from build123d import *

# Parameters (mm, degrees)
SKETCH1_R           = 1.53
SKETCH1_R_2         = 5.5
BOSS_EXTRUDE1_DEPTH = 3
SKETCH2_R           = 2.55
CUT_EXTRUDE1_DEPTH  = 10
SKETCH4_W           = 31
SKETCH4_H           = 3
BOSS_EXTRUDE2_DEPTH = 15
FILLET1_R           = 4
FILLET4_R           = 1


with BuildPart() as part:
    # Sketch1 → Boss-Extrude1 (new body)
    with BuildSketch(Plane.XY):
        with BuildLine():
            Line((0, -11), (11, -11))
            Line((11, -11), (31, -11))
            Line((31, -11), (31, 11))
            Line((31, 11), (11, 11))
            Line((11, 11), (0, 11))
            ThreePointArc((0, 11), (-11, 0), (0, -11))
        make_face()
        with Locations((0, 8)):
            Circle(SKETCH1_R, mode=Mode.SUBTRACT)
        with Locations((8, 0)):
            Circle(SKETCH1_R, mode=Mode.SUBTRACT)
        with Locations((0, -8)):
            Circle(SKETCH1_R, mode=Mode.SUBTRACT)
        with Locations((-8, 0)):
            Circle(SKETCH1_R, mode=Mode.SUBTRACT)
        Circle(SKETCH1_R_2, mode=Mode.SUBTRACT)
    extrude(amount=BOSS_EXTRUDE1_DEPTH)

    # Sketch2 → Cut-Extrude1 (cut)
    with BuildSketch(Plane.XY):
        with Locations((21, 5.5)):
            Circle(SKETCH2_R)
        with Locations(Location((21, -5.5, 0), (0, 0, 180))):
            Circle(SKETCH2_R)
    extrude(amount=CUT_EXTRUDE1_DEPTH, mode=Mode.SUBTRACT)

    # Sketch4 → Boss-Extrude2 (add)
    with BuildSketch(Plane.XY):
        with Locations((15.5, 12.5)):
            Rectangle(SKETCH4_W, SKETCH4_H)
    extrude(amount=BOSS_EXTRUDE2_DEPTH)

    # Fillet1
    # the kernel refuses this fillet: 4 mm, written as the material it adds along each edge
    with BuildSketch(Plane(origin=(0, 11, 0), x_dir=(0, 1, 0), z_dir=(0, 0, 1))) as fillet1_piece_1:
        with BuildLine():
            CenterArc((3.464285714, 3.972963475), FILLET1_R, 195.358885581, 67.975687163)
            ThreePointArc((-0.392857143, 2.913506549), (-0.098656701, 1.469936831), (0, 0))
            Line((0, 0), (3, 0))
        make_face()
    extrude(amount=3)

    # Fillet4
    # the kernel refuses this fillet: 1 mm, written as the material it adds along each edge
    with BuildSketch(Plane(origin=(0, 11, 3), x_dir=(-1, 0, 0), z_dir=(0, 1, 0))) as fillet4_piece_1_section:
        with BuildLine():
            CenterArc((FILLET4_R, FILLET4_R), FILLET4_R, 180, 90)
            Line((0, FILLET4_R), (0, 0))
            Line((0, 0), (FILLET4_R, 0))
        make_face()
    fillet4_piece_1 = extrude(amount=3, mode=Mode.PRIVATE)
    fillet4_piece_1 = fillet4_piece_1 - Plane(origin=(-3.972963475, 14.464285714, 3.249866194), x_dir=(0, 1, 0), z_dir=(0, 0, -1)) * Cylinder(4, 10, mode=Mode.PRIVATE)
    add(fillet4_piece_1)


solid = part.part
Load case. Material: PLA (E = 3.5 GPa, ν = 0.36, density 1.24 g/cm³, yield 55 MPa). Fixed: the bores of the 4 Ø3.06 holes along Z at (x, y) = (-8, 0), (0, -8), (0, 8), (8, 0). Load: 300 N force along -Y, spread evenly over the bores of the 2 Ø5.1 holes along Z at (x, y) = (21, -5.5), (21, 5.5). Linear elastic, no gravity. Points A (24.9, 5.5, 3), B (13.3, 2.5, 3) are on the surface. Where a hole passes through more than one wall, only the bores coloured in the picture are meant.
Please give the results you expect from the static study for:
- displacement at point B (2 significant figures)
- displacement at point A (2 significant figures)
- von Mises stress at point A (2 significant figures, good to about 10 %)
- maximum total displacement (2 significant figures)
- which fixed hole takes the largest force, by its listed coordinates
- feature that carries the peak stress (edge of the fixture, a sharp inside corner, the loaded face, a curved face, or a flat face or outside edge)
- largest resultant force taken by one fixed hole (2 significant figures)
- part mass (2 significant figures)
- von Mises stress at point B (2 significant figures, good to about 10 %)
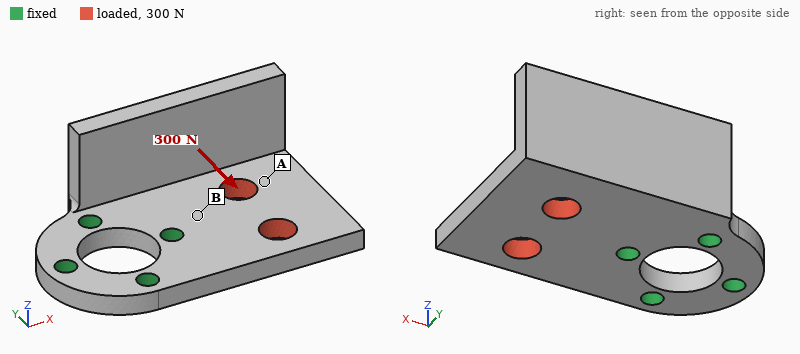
0.039 mm
0.13 mm
3.6 MPa
0.17 mm
(8, 0)
edge of the fixture
340 N
4.4 g
10 MPa
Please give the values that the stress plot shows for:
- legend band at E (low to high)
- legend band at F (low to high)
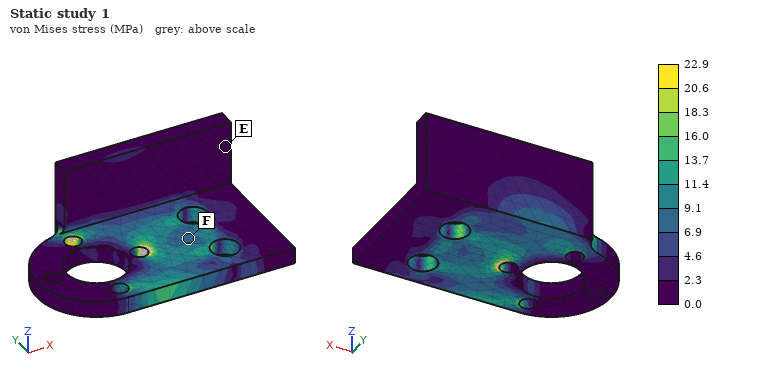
0.0 to 2.3 MPa
6.9 to 9.1 MPa
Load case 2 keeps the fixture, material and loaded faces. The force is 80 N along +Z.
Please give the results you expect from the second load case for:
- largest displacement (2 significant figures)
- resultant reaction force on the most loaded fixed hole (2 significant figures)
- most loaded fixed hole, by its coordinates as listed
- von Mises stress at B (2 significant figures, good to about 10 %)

0.55 mm
110 N
(8, 0)
13 MPa
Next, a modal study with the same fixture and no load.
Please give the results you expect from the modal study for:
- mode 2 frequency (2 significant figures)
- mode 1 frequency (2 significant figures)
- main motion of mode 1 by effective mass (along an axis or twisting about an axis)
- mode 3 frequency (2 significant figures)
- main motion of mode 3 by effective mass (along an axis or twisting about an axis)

2000 Hz
1200 Hz
along Z
3300 Hz
along Y
